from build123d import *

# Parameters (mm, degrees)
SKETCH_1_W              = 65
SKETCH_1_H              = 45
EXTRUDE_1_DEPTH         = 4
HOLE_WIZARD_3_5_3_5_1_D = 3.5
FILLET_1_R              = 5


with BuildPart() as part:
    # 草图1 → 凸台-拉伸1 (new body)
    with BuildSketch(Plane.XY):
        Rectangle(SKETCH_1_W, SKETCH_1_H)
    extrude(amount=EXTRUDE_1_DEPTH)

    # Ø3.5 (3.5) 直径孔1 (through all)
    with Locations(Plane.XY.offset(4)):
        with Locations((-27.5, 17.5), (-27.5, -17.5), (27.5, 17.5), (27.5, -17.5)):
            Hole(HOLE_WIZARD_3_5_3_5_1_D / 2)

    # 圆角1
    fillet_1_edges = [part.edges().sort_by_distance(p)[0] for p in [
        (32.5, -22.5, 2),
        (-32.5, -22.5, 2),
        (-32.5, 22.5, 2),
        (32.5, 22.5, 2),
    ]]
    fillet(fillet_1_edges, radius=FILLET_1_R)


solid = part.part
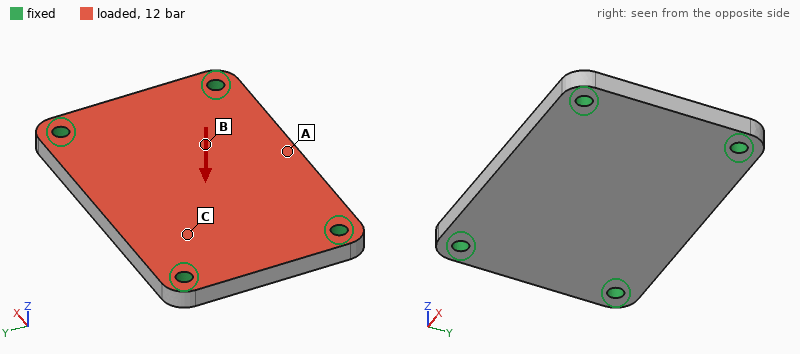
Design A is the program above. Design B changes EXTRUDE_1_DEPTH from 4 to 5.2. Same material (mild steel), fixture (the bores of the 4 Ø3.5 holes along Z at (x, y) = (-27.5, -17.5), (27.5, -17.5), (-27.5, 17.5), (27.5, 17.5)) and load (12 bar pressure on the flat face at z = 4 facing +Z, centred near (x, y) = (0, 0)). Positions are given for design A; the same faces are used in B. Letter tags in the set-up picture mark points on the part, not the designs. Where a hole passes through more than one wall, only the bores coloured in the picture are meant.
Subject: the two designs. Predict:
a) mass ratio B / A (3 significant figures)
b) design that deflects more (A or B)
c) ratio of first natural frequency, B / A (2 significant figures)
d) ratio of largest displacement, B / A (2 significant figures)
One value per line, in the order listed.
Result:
1.30
A
1.2
0.49
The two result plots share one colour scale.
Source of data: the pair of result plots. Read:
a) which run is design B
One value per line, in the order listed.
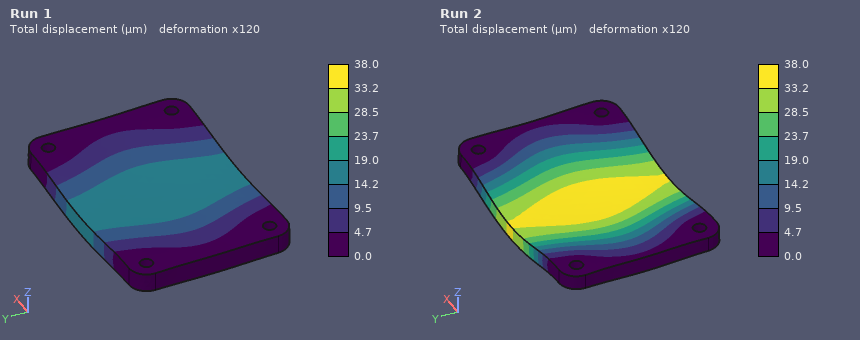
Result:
Run 1
